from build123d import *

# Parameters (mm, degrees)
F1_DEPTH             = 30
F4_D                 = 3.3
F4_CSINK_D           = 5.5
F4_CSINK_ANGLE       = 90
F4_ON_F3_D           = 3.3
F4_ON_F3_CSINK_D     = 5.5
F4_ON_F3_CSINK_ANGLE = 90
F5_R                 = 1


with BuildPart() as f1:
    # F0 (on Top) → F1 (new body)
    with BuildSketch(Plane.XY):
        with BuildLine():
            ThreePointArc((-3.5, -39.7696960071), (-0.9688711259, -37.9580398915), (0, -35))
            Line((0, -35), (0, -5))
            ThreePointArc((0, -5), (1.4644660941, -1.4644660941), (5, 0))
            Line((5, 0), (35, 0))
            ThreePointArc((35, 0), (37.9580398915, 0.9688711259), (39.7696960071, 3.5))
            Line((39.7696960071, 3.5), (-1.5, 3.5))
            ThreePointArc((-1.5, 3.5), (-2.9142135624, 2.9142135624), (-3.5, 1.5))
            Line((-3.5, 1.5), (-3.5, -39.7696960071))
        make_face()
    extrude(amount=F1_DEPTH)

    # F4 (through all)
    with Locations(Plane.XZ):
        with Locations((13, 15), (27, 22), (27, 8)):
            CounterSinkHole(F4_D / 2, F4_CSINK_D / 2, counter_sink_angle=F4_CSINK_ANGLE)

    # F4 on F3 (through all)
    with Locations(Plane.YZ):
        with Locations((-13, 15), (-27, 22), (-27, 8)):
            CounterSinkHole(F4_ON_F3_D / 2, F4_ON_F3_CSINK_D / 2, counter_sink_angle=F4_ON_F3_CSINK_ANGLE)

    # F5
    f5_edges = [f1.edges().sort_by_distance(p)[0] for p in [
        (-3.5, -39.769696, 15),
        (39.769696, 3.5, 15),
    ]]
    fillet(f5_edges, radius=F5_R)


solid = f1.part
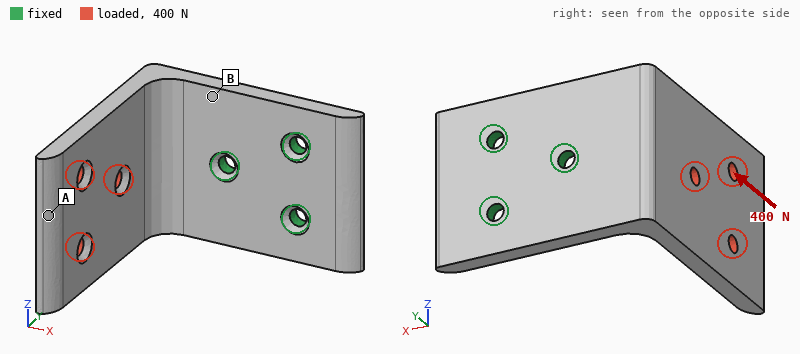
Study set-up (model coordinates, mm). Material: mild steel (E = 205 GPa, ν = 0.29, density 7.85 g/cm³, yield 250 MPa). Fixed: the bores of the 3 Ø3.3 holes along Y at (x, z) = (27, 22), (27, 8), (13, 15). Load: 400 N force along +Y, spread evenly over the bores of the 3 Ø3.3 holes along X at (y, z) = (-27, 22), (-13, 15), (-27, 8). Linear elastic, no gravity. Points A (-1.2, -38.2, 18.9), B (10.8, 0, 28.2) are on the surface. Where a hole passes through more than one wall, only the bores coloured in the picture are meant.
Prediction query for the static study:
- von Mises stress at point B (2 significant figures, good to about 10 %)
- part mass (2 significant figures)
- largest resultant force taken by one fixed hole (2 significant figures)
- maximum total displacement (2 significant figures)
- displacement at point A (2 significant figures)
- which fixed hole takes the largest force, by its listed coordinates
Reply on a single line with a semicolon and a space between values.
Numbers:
57 MPa; 65 g; 690 N; 0.11 mm; 0.11 mm; (13, 15)
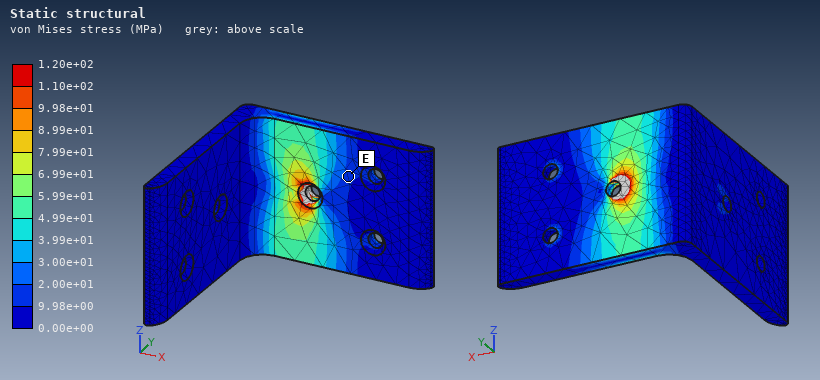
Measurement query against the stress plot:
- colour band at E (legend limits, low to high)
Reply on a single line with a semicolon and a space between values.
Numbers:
9.98e+00 to 2.00e+01 MPa
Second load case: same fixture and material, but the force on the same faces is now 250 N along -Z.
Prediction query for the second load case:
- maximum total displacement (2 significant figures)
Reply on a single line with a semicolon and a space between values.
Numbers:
0.10 mm
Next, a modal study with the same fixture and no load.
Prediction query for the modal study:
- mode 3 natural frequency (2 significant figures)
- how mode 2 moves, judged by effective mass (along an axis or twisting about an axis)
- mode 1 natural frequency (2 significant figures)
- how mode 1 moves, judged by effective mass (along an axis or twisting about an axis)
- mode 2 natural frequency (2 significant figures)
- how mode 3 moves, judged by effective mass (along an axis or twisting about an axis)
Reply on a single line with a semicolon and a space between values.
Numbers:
4400 Hz; along Z; 1200 Hz; along X; 1800 Hz; along Y
